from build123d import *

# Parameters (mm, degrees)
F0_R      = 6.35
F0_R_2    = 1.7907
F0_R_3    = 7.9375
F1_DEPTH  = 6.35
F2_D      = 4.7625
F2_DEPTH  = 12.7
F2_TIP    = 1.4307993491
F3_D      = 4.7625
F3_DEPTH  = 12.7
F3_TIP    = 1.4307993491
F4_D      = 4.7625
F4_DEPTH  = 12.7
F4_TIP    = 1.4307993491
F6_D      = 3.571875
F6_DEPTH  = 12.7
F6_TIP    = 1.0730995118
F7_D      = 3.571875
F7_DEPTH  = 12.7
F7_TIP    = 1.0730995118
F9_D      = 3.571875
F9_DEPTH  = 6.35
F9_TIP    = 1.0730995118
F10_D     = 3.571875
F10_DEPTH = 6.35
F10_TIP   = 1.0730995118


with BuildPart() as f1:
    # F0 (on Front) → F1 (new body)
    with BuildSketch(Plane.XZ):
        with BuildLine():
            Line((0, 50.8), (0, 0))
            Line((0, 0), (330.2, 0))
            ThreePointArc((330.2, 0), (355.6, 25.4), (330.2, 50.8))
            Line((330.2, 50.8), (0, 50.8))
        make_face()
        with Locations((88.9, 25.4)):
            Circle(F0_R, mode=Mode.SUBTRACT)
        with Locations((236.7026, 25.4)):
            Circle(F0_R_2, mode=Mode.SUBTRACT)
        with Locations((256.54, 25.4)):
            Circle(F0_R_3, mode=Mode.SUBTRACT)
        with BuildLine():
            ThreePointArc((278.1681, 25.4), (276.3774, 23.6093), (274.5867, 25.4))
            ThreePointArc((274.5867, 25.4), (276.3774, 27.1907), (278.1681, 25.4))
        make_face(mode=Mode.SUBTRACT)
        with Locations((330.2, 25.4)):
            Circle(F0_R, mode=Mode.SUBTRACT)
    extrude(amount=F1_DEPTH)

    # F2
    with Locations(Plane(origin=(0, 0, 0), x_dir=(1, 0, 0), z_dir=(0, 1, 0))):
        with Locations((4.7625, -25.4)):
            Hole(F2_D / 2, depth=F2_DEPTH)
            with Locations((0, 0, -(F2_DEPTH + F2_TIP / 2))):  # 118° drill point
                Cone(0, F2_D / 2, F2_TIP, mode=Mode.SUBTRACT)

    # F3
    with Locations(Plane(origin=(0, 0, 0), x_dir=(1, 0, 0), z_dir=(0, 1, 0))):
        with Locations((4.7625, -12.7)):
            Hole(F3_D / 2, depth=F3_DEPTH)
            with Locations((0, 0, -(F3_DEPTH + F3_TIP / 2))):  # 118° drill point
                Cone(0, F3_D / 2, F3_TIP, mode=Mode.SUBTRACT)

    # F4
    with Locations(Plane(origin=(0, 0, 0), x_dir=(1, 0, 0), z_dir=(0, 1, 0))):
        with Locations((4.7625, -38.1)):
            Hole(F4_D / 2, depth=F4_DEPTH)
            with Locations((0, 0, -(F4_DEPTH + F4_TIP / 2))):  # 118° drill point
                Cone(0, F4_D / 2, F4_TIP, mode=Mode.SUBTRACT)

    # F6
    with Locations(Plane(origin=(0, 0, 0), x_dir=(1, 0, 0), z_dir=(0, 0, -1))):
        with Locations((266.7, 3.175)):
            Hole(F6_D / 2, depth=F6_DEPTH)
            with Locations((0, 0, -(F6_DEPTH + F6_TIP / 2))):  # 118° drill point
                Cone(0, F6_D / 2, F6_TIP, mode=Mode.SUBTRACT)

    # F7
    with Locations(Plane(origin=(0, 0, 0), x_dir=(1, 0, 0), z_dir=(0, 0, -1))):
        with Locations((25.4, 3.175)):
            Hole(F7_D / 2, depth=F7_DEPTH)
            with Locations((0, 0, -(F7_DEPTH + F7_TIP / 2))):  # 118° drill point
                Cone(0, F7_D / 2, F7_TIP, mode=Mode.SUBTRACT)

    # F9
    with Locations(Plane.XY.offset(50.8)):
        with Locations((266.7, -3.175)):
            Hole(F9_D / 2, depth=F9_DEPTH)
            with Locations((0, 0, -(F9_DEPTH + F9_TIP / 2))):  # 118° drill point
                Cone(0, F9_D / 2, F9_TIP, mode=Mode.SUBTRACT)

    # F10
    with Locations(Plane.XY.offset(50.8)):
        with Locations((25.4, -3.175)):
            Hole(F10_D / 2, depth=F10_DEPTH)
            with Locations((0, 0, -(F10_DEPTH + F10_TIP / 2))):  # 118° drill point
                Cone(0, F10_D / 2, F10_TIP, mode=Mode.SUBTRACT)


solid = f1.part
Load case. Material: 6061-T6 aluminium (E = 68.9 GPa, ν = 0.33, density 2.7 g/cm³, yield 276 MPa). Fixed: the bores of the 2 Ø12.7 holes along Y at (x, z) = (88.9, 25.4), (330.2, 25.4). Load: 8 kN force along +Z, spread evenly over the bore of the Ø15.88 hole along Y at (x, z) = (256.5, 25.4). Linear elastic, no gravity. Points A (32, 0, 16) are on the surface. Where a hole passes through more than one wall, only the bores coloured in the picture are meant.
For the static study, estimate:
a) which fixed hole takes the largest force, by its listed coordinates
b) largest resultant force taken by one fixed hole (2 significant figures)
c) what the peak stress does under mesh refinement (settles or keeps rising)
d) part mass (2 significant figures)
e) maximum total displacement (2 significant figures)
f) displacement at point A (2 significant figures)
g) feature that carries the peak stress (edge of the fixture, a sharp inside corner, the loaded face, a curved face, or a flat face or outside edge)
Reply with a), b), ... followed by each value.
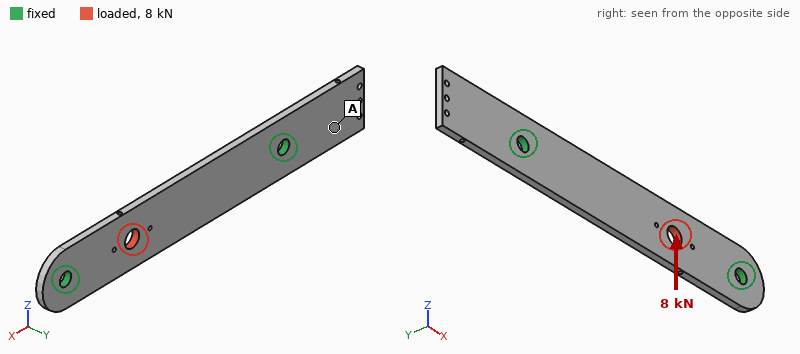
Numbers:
a) (330.2, 25.4)
b) 5.9 kN
c) keeps rising
d) 290 g
e) 0.23 mm
f) 0.062 mm
g) a sharp inside corner
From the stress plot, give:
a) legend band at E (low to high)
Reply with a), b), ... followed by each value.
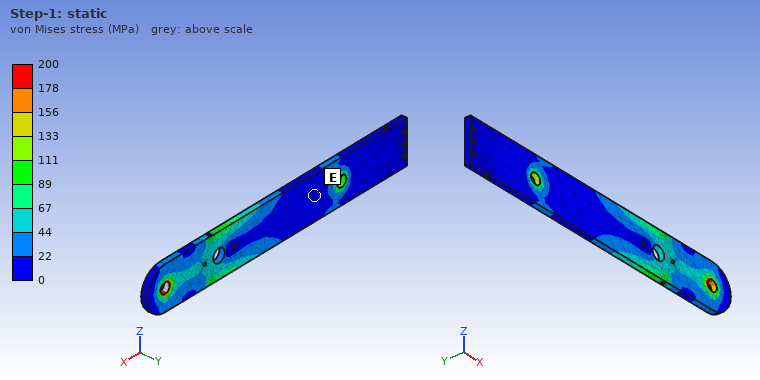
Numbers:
a) 0 to 22 MPa
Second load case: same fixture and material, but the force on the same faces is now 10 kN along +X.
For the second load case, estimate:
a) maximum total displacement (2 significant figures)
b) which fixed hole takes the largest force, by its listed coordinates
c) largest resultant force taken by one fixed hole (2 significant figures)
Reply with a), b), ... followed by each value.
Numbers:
a) 30 µm
b) (330.2, 25.4)
c) 6.7 kN
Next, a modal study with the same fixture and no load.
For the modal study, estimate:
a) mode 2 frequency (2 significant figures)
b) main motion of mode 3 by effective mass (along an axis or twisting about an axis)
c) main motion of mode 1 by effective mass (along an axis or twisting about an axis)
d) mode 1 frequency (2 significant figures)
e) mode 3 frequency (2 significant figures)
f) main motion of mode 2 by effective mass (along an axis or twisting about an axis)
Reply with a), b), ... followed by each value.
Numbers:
a) 730 Hz
b) twisting about X
c) along Y
d) 600 Hz
e) 1600 Hz
f) along Y
